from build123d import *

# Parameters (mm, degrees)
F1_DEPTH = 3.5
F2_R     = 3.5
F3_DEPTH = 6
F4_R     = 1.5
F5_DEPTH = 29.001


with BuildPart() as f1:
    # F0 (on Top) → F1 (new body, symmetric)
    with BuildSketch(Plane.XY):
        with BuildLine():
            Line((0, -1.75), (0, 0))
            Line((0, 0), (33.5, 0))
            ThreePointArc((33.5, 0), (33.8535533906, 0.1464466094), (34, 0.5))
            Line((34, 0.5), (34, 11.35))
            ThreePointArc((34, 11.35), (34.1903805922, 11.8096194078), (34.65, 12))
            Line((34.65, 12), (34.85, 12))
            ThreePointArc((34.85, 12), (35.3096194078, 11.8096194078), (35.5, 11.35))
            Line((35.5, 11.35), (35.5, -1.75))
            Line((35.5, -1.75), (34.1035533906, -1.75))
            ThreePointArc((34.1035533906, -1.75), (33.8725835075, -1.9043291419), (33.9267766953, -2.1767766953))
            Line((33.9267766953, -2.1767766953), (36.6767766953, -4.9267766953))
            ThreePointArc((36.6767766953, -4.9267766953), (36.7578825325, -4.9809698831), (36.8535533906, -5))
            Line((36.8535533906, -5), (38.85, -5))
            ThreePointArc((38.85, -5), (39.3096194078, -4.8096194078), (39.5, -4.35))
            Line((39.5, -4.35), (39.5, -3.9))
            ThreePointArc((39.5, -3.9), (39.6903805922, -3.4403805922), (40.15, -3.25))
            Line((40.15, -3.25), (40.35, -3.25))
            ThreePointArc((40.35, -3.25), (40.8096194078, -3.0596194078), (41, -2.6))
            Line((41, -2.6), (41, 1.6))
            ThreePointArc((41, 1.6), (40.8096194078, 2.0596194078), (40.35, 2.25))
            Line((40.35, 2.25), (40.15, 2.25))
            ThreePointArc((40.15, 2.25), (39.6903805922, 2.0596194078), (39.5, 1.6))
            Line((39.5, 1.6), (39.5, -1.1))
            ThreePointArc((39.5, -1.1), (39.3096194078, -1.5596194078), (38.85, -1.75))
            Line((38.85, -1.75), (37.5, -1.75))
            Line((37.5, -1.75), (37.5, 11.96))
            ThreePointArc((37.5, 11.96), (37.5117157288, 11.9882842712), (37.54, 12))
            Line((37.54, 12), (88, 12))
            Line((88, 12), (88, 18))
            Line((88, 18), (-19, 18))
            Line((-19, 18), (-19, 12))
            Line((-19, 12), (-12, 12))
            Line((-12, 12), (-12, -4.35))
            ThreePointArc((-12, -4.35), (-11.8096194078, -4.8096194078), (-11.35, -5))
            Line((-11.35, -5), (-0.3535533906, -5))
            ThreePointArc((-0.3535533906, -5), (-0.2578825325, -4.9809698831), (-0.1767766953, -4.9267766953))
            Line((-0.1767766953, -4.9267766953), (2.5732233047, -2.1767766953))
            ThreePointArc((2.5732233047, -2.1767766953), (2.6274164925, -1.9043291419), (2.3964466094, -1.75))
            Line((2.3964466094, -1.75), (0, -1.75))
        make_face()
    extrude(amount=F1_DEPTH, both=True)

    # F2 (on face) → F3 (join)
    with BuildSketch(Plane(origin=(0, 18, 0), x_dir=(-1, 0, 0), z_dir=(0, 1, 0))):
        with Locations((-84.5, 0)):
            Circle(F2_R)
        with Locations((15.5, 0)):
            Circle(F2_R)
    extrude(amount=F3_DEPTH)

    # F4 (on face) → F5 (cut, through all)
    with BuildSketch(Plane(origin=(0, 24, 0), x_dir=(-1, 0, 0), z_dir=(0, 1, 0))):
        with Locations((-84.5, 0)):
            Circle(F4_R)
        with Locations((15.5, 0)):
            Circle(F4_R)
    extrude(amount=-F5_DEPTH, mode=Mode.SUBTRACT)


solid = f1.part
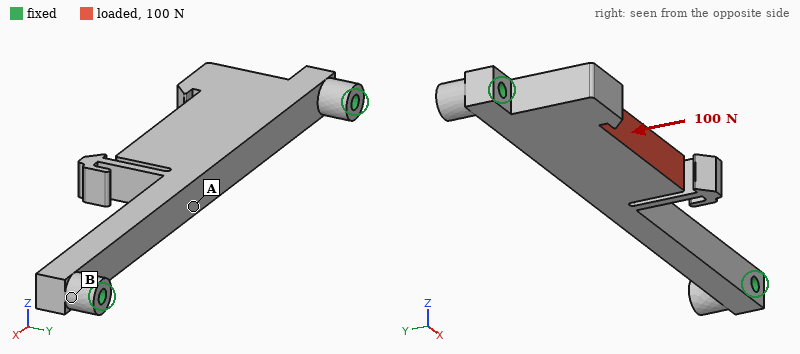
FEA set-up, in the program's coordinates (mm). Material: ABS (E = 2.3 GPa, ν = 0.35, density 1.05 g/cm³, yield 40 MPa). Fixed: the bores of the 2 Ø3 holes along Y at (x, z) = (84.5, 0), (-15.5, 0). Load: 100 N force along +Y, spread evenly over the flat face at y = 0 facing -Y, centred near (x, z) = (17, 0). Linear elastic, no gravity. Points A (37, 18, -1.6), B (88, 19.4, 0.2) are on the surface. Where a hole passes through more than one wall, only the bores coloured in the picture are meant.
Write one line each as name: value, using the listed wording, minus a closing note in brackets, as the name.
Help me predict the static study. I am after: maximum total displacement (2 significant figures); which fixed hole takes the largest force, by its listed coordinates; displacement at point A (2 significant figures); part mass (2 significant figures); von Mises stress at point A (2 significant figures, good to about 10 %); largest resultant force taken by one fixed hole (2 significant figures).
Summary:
maximum total displacement: 0.81 mm
which fixed hole takes the largest force, by its listed coordinates: (-15.5, 0)
displacement at point A: 0.77 mm
part mass: 9.9 g
von Mises stress at point A: 14 MPa
largest resultant force taken by one fixed hole: 76 N
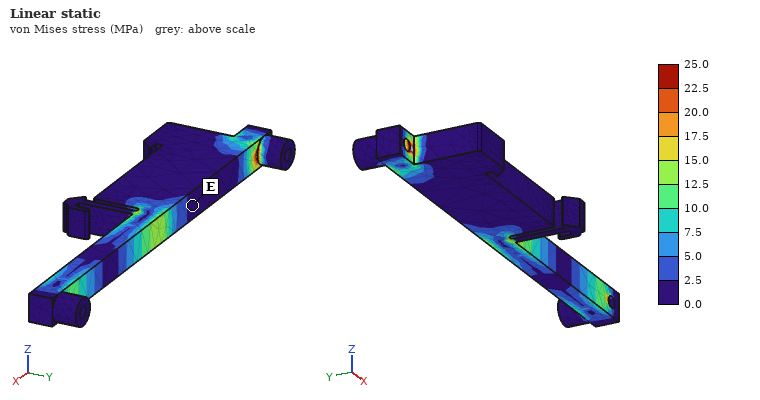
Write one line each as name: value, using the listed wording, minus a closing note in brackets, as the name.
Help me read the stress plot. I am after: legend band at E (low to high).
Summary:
legend band at E: 0.0 to 2.5 MPa
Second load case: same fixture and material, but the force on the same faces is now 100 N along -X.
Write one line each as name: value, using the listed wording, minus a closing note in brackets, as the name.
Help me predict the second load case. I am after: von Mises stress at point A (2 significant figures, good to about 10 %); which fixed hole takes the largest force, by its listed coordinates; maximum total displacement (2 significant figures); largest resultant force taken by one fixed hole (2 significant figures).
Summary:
von Mises stress at point A: 7.2 MPa
which fixed hole takes the largest force, by its listed coordinates: (-15.5, 0)
maximum total displacement: 0.42 mm
largest resultant force taken by one fixed hole: 79 N
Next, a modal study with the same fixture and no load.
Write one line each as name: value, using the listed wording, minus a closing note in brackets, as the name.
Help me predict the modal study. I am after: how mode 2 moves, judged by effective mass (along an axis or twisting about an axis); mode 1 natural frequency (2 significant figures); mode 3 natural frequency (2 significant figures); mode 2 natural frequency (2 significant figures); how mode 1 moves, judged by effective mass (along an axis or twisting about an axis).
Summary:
how mode 2 moves, judged by effective mass: along Y
mode 1 natural frequency: 710 Hz
mode 3 natural frequency: 1100 Hz
mode 2 natural frequency: 750 Hz
how mode 1 moves, judged by effective mass: along Z
